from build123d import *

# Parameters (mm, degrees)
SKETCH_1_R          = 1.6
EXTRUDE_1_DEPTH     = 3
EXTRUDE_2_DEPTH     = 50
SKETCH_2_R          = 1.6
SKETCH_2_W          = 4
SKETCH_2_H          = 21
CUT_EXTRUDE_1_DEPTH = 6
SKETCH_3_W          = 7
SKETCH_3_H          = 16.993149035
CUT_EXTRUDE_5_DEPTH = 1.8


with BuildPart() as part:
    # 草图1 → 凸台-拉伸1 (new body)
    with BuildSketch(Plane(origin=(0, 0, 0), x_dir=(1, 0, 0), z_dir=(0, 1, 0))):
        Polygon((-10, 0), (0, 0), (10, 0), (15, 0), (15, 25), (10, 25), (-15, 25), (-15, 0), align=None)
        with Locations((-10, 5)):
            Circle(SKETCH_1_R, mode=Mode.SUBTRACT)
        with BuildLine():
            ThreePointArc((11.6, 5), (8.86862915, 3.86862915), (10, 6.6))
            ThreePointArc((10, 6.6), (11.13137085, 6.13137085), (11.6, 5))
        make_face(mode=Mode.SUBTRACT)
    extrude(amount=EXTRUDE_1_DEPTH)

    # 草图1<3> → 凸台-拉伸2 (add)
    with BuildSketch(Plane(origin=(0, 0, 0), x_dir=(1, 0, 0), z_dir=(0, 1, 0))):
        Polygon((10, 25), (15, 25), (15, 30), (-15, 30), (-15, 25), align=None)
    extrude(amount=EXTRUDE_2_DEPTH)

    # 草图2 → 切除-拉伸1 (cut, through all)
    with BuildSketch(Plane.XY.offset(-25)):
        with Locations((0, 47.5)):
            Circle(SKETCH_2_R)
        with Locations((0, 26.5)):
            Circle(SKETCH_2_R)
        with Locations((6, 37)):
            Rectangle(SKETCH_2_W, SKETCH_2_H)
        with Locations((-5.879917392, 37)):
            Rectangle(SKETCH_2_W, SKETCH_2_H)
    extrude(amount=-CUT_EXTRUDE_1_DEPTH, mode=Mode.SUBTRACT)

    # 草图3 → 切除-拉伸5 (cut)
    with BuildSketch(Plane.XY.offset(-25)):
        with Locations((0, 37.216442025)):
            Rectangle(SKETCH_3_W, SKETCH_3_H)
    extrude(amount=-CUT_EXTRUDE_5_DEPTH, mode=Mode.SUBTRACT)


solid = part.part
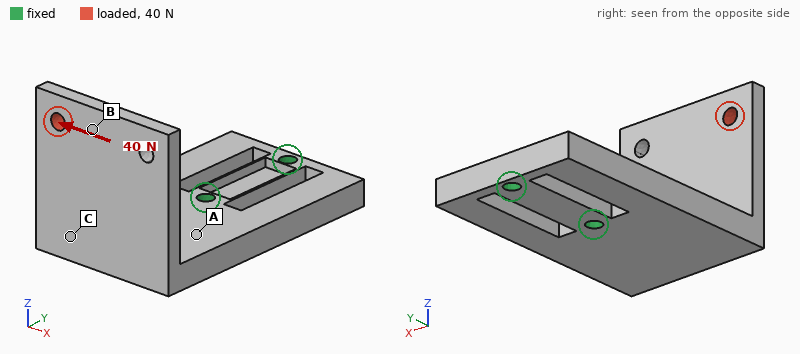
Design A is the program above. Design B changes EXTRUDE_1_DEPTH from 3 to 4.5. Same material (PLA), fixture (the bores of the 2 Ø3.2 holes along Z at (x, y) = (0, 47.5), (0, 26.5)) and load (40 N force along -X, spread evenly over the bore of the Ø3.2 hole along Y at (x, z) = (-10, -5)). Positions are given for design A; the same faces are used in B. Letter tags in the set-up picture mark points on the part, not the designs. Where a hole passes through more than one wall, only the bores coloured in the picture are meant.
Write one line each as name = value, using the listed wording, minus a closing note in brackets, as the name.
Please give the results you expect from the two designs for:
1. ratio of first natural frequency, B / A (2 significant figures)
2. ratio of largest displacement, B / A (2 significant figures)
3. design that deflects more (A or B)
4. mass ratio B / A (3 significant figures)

ratio of first natural frequency, B / A = 0.91
ratio of largest displacement, B / A = 0.90
design that deflects more = A
mass ratio B / A = 1.13
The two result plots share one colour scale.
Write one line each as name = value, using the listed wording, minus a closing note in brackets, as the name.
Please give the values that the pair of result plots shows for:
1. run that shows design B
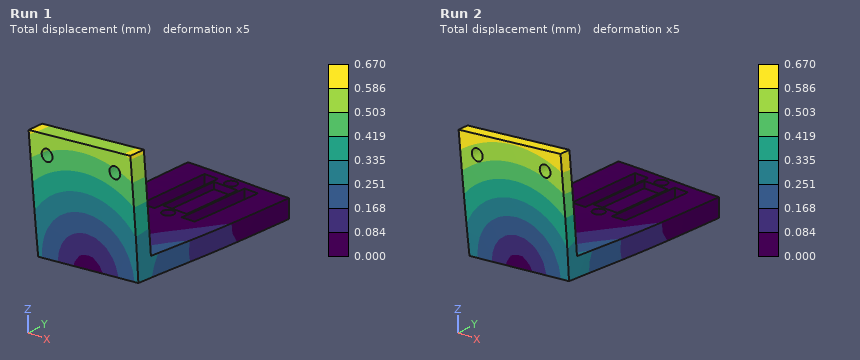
run that shows design B = Run 1
